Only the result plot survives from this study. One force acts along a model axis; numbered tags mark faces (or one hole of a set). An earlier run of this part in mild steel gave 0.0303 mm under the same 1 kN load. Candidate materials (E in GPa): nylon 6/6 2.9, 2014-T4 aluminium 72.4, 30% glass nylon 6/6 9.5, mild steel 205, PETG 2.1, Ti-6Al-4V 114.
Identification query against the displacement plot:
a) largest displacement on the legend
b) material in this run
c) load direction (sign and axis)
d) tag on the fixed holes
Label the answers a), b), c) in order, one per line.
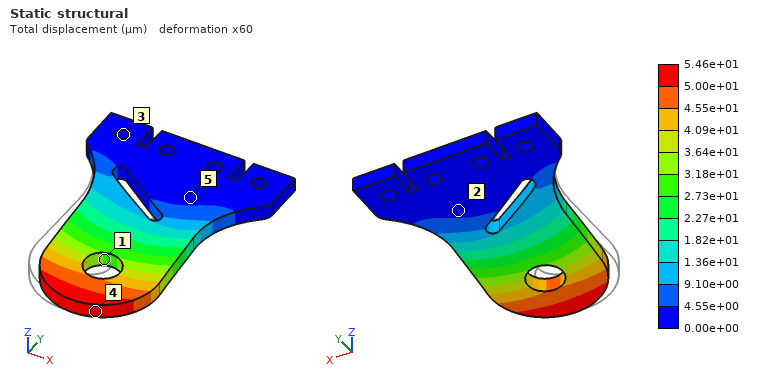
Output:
a) 5.46e+01 µm
b) Ti-6Al-4V
c) +X
d) 3
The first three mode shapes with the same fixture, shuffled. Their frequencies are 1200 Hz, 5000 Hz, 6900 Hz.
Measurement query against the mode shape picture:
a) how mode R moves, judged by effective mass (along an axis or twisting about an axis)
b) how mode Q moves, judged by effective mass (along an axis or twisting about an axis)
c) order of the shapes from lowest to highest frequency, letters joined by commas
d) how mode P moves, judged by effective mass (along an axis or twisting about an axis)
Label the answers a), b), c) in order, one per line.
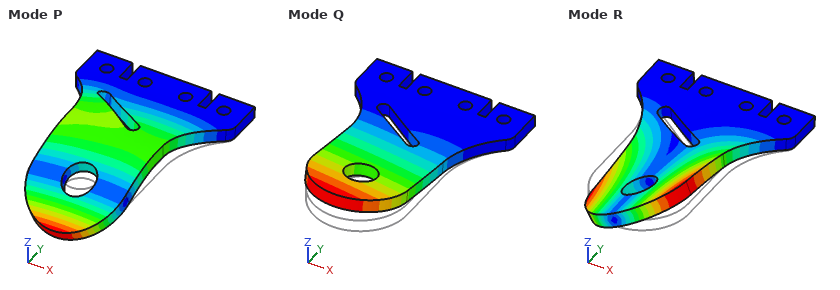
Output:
a) twisting about Y
b) along Z
c) Q, R, P
d) along Z
